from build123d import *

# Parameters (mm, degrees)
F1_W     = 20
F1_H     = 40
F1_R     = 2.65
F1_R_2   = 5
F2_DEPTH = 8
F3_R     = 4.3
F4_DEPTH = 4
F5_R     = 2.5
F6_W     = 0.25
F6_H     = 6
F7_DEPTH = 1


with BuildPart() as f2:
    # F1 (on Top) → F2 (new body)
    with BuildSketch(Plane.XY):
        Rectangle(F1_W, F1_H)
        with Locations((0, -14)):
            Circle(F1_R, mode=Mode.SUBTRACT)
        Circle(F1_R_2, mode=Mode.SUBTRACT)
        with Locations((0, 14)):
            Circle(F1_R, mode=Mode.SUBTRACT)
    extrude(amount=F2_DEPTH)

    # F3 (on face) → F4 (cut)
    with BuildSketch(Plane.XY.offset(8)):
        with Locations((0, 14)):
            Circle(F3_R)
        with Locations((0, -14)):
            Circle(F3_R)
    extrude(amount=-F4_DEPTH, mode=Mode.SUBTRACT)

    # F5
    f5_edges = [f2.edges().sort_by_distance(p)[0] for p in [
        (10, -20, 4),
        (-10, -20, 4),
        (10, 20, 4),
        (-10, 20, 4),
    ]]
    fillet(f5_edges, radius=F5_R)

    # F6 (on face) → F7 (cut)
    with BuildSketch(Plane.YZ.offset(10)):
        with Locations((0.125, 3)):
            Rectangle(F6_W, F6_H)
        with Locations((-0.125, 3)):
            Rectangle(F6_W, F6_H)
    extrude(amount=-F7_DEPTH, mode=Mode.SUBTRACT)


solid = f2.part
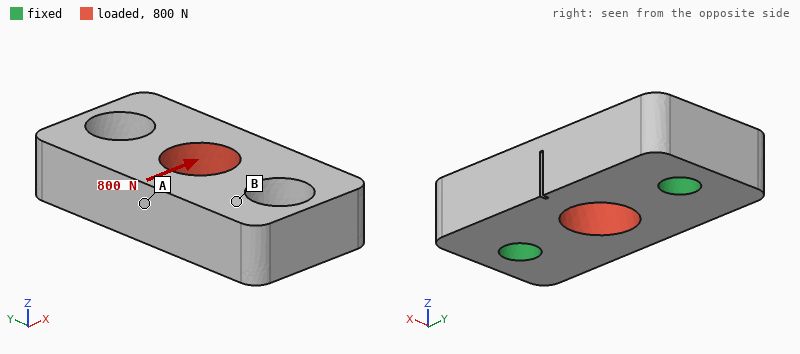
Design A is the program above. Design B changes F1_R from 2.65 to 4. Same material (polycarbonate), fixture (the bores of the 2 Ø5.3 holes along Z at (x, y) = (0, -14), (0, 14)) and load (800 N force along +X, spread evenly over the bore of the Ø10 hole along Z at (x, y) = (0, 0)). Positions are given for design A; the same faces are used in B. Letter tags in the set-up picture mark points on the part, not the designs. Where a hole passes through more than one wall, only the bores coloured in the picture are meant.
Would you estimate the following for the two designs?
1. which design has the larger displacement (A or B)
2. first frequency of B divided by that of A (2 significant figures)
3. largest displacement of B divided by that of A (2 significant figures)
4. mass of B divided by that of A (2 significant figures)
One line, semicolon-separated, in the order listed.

A; 1.4; 0.63; 0.96
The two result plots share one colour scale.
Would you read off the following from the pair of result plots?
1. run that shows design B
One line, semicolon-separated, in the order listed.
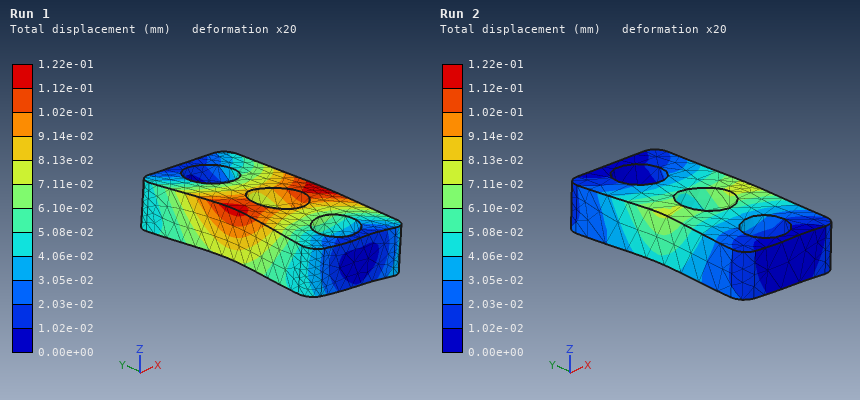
Run 2
